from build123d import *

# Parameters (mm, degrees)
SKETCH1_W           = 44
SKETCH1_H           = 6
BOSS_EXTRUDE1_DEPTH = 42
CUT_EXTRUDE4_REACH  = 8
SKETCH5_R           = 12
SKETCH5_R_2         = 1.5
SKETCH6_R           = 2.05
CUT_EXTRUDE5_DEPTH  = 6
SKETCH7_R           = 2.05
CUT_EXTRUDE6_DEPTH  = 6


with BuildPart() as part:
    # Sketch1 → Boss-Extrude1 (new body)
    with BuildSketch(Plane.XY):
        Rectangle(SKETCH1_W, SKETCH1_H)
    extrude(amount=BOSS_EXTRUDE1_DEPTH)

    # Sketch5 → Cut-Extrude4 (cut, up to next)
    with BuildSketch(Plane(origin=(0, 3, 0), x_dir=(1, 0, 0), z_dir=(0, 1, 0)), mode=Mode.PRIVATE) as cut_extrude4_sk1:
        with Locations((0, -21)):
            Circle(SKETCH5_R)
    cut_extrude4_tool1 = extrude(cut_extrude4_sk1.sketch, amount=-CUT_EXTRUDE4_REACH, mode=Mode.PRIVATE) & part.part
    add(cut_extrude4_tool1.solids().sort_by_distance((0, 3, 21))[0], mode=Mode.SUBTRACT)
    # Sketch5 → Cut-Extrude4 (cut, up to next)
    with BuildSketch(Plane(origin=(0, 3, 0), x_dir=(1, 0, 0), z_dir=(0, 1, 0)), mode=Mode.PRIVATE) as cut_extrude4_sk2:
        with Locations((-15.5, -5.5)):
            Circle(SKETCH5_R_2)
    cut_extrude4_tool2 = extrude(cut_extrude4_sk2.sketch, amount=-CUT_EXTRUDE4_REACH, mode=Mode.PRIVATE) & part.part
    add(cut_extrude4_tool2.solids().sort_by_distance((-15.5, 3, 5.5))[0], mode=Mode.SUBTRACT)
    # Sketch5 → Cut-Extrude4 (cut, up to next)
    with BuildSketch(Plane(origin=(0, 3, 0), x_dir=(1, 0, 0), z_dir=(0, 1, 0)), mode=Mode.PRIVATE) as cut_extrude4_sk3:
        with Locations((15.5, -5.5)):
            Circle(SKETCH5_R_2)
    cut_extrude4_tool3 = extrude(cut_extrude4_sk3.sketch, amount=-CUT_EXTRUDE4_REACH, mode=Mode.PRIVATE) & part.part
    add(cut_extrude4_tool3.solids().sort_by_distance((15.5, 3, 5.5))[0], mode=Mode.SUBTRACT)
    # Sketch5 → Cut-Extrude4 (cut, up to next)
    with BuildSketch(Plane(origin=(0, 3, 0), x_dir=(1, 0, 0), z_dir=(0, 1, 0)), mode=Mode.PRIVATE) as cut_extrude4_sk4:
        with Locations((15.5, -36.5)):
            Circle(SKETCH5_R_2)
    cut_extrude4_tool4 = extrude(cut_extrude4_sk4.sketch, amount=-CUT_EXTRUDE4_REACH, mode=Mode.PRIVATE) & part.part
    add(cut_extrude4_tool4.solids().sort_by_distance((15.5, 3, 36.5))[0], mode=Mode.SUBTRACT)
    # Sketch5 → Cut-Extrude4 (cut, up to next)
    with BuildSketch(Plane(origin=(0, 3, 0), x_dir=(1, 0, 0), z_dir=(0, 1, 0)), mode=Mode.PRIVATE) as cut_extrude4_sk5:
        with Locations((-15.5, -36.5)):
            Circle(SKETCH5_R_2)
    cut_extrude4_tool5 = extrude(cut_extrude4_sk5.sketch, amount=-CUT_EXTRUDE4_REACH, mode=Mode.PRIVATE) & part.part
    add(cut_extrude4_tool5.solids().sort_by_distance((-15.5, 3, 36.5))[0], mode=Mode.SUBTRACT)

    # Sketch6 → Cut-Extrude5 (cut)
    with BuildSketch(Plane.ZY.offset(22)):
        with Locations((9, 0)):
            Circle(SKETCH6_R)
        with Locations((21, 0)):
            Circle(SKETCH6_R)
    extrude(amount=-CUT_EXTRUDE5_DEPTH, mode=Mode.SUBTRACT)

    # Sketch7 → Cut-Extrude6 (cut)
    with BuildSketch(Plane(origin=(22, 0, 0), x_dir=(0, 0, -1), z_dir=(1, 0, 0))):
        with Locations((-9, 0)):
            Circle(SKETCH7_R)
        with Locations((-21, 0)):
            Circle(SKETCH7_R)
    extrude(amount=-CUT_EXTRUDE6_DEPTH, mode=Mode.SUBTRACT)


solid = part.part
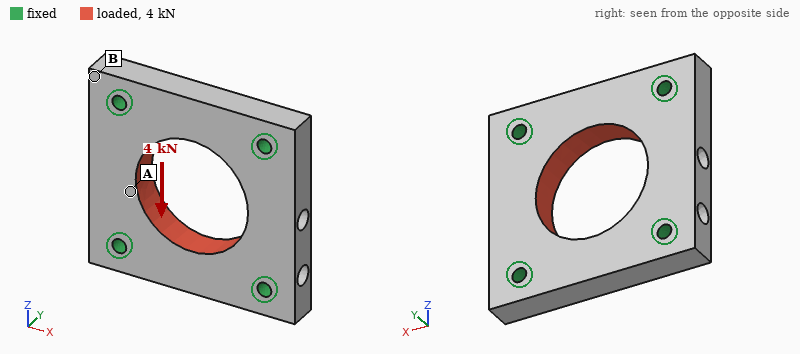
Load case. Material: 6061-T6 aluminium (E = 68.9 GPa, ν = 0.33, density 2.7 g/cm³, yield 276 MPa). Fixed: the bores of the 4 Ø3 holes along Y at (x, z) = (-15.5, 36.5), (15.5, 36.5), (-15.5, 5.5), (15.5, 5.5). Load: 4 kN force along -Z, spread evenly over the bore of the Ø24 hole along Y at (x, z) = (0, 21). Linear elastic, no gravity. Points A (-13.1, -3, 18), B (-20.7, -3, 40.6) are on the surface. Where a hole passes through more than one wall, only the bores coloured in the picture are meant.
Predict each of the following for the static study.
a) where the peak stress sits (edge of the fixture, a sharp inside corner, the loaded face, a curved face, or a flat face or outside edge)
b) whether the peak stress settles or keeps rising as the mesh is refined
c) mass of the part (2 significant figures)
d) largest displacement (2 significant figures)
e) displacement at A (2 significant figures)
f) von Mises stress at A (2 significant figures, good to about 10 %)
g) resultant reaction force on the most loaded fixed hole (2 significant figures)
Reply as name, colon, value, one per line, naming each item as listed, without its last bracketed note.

where the peak stress sits: edge of the fixture
whether the peak stress settles or keeps rising as the mesh is refined: keeps rising
mass of the part: 21 g
largest displacement: 7.1 µm
displacement at A: 2.5 µm
von Mises stress at A: 16 MPa
resultant reaction force on the most loaded fixed hole: 1.1 kN
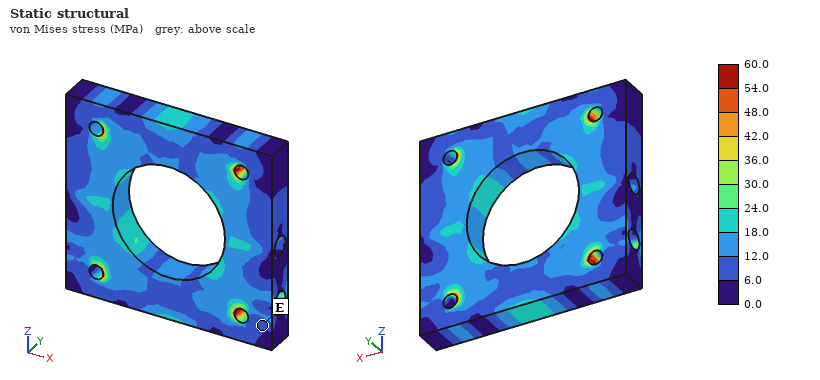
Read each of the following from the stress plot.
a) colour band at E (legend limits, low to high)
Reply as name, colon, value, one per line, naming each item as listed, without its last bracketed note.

colour band at E: 6.0 to 12.0 MPa
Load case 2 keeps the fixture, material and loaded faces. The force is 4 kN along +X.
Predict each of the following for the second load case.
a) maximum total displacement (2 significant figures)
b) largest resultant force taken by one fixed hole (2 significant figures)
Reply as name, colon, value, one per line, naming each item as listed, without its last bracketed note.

maximum total displacement: 7.4 µm
largest resultant force taken by one fixed hole: 1.0 kN
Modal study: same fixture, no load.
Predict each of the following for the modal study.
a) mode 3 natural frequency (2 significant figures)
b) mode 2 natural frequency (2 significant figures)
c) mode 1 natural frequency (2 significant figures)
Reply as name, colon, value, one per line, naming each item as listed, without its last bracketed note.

mode 3 natural frequency: 26 kHz
mode 2 natural frequency: 25 kHz
mode 1 natural frequency: 25 kHz
